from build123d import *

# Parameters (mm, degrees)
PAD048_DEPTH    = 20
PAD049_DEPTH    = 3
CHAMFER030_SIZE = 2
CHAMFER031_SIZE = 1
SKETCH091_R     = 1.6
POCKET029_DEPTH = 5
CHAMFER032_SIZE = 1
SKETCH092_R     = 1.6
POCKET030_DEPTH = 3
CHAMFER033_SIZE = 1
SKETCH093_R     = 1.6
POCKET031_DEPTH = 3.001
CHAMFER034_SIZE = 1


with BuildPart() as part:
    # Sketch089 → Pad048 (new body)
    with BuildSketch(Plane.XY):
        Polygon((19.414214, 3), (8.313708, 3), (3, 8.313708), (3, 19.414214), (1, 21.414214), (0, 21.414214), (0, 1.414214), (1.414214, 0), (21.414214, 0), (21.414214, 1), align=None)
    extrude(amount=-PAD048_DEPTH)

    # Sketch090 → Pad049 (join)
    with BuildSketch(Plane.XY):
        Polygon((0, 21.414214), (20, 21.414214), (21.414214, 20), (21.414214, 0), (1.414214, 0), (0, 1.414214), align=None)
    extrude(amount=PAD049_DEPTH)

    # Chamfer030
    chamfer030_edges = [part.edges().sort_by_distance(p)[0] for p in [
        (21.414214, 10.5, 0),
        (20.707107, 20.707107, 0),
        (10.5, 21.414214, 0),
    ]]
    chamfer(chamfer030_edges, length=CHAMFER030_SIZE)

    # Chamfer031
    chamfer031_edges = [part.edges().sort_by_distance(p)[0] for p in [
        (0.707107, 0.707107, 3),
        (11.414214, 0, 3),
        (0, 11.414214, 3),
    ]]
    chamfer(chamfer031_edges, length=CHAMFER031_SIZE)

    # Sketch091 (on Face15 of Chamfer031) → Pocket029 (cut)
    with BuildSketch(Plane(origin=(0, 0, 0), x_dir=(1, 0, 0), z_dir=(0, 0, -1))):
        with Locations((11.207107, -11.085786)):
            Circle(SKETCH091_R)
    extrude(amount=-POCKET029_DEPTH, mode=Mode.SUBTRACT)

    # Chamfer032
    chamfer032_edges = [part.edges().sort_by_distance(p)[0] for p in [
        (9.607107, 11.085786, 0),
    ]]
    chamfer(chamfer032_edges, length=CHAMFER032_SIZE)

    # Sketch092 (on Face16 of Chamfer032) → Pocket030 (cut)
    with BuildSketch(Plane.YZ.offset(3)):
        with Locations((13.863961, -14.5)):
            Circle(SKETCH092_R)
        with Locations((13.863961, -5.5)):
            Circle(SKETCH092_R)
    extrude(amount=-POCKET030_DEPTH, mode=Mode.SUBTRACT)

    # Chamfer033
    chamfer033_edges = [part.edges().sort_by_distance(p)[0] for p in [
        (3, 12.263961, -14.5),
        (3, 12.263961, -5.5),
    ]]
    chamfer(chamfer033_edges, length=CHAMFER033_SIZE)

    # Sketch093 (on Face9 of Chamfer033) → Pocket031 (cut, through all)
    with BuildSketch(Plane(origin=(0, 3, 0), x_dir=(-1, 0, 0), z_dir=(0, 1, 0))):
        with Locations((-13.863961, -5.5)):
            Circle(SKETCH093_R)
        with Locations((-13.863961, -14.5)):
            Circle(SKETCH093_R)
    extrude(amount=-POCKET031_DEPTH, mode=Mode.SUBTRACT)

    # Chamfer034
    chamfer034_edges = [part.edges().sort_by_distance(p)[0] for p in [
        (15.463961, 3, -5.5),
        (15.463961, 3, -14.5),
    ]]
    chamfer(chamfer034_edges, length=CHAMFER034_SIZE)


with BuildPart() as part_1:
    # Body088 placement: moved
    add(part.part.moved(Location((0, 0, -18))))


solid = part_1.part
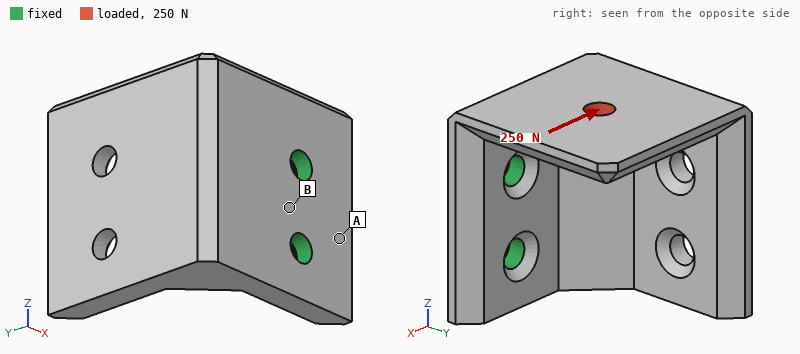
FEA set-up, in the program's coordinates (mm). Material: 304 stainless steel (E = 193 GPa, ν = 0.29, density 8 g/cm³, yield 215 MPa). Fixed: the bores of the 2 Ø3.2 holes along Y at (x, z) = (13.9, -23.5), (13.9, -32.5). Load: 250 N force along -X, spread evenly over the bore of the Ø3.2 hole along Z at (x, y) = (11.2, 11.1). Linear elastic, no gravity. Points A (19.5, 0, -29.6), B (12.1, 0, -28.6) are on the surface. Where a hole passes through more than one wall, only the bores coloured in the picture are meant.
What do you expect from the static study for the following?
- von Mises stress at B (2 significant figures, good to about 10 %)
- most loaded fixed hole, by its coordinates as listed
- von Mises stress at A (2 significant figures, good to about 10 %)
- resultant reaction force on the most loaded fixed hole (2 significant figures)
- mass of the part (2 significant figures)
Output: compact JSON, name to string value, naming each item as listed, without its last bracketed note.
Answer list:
{"von Mises stress at B": "36 MPa", "most loaded fixed hole, by its coordinates as listed": "(13.9, -23.5)", "von Mises stress at A": "18 MPa", "resultant reaction force on the most loaded fixed hole": "370 N", "mass of the part": "30 g"}
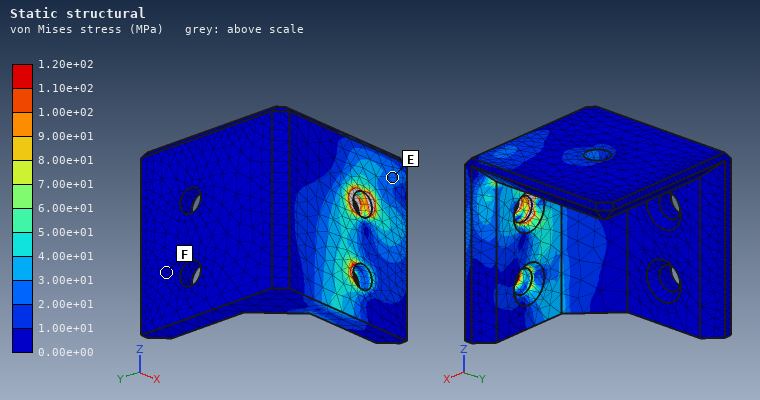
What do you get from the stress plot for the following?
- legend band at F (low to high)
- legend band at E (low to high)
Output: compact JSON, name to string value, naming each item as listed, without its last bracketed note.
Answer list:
{"legend band at F": "0.00e+00 to 1.00e+01 MPa", "legend band at E": "2.00e+01 to 3.00e+01 MPa"}
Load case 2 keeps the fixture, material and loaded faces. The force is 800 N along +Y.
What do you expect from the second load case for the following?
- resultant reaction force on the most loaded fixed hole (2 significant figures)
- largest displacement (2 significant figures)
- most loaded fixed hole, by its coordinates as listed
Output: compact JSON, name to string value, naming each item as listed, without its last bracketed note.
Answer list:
{"resultant reaction force on the most loaded fixed hole": "1.1 kN", "largest displacement": "44 µm", "most loaded fixed hole, by its coordinates as listed": "(13.9, -23.5)"}
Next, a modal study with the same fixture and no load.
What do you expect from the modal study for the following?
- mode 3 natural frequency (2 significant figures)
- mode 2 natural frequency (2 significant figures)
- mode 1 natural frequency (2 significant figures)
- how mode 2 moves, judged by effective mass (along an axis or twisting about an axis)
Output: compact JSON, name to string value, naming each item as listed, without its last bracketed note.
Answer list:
{"mode 3 natural frequency": "12 kHz", "mode 2 natural frequency": "5400 Hz", "mode 1 natural frequency": "3500 Hz", "how mode 2 moves, judged by effective mass": "along Z"}
